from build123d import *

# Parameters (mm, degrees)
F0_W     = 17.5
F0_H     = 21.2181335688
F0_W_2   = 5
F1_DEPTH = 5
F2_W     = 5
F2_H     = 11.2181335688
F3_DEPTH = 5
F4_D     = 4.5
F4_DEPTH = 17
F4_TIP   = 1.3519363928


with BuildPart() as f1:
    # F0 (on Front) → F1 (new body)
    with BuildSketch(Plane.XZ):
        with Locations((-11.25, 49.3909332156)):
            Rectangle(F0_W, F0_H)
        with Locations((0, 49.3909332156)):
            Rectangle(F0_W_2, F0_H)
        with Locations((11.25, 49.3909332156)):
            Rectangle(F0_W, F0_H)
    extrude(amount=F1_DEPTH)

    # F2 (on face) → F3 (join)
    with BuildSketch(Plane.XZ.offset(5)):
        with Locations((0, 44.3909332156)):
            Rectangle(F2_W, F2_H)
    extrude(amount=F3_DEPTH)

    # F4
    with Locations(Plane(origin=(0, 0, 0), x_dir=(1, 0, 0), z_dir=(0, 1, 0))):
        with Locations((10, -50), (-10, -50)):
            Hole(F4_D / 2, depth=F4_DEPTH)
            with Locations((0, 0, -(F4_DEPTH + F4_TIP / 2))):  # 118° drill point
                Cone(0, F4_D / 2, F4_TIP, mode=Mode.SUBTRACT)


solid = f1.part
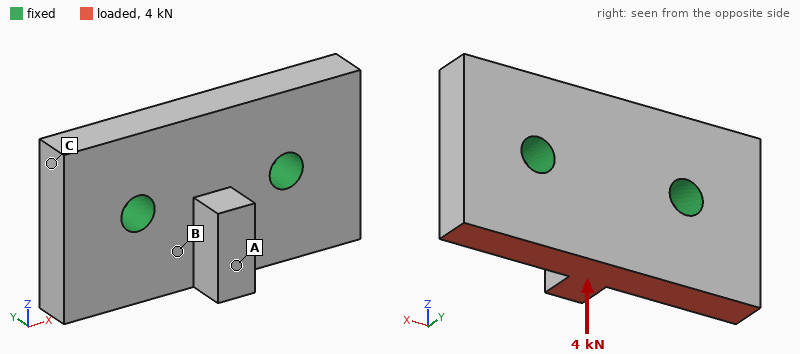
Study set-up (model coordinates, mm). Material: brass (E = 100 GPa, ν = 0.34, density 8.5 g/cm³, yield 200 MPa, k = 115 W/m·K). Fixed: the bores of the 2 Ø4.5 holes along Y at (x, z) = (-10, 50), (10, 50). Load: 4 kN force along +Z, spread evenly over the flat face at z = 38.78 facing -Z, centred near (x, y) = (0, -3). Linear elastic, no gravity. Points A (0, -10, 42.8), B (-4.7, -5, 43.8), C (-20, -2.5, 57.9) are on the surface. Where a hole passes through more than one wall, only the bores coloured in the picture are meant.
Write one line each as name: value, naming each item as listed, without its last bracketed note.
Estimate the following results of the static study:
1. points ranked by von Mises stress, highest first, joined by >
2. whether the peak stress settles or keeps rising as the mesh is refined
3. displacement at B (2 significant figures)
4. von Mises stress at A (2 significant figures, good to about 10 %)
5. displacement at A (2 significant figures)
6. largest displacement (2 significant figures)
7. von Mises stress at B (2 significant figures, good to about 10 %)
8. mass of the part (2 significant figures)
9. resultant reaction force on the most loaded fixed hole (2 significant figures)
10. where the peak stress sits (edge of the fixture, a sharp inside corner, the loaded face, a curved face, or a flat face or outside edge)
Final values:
points ranked by von Mises stress, highest first, joined by >: B > A > C
whether the peak stress settles or keeps rising as the mesh is refined: keeps rising
displacement at B: 3.2 µm
von Mises stress at A: 15 MPa
displacement at A: 6.9 µm
largest displacement: 8.5 µm
von Mises stress at B: 30 MPa
mass of the part: 37 g
resultant reaction force on the most loaded fixed hole: 2.0 kN
where the peak stress sits: edge of the fixture
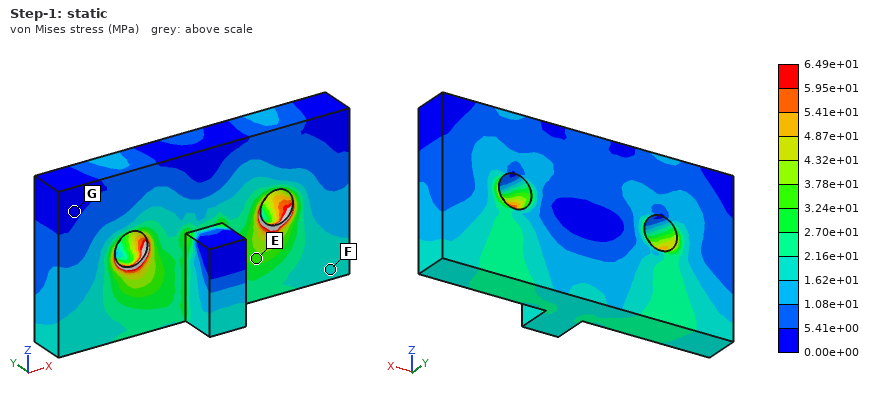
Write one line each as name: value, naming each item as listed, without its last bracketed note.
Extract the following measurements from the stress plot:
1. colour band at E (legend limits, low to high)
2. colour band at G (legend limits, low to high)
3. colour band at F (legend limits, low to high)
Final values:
colour band at E: 3.24e+01 to 3.78e+01 MPa
colour band at G: 0.00e+00 to 5.41e+00 MPa
colour band at F: 1.62e+01 to 2.16e+01 MPa
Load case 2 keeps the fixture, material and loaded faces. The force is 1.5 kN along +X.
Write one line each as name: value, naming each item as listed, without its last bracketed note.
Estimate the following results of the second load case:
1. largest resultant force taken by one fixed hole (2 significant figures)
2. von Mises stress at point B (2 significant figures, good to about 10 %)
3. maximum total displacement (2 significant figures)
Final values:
largest resultant force taken by one fixed hole: 1000 N
von Mises stress at point B: 24 MPa
maximum total displacement: 5.6 µm
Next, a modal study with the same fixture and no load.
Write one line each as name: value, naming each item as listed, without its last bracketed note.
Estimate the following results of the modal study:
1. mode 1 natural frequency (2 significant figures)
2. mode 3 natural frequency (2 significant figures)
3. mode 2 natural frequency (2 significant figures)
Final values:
mode 1 natural frequency: 17 kHz
mode 3 natural frequency: 21 kHz
mode 2 natural frequency: 20 kHz
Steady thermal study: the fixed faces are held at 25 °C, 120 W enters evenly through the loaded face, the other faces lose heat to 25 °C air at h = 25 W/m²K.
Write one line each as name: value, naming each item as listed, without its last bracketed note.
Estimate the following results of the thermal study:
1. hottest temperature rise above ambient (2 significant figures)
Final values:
hottest temperature rise above ambient: 67 K
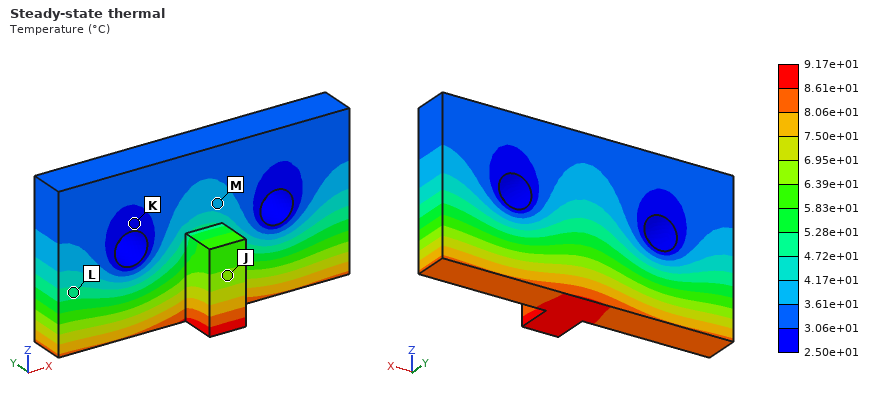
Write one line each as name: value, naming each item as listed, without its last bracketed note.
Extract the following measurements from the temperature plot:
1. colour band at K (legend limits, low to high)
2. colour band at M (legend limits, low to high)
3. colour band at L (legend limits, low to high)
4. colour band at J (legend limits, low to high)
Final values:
colour band at K: 2.50e+01 to 3.06e+01 °C
colour band at M: 3.61e+01 to 4.17e+01 °C
colour band at L: 4.72e+01 to 5.28e+01 °C
colour band at J: 6.39e+01 to 6.95e+01 °C
